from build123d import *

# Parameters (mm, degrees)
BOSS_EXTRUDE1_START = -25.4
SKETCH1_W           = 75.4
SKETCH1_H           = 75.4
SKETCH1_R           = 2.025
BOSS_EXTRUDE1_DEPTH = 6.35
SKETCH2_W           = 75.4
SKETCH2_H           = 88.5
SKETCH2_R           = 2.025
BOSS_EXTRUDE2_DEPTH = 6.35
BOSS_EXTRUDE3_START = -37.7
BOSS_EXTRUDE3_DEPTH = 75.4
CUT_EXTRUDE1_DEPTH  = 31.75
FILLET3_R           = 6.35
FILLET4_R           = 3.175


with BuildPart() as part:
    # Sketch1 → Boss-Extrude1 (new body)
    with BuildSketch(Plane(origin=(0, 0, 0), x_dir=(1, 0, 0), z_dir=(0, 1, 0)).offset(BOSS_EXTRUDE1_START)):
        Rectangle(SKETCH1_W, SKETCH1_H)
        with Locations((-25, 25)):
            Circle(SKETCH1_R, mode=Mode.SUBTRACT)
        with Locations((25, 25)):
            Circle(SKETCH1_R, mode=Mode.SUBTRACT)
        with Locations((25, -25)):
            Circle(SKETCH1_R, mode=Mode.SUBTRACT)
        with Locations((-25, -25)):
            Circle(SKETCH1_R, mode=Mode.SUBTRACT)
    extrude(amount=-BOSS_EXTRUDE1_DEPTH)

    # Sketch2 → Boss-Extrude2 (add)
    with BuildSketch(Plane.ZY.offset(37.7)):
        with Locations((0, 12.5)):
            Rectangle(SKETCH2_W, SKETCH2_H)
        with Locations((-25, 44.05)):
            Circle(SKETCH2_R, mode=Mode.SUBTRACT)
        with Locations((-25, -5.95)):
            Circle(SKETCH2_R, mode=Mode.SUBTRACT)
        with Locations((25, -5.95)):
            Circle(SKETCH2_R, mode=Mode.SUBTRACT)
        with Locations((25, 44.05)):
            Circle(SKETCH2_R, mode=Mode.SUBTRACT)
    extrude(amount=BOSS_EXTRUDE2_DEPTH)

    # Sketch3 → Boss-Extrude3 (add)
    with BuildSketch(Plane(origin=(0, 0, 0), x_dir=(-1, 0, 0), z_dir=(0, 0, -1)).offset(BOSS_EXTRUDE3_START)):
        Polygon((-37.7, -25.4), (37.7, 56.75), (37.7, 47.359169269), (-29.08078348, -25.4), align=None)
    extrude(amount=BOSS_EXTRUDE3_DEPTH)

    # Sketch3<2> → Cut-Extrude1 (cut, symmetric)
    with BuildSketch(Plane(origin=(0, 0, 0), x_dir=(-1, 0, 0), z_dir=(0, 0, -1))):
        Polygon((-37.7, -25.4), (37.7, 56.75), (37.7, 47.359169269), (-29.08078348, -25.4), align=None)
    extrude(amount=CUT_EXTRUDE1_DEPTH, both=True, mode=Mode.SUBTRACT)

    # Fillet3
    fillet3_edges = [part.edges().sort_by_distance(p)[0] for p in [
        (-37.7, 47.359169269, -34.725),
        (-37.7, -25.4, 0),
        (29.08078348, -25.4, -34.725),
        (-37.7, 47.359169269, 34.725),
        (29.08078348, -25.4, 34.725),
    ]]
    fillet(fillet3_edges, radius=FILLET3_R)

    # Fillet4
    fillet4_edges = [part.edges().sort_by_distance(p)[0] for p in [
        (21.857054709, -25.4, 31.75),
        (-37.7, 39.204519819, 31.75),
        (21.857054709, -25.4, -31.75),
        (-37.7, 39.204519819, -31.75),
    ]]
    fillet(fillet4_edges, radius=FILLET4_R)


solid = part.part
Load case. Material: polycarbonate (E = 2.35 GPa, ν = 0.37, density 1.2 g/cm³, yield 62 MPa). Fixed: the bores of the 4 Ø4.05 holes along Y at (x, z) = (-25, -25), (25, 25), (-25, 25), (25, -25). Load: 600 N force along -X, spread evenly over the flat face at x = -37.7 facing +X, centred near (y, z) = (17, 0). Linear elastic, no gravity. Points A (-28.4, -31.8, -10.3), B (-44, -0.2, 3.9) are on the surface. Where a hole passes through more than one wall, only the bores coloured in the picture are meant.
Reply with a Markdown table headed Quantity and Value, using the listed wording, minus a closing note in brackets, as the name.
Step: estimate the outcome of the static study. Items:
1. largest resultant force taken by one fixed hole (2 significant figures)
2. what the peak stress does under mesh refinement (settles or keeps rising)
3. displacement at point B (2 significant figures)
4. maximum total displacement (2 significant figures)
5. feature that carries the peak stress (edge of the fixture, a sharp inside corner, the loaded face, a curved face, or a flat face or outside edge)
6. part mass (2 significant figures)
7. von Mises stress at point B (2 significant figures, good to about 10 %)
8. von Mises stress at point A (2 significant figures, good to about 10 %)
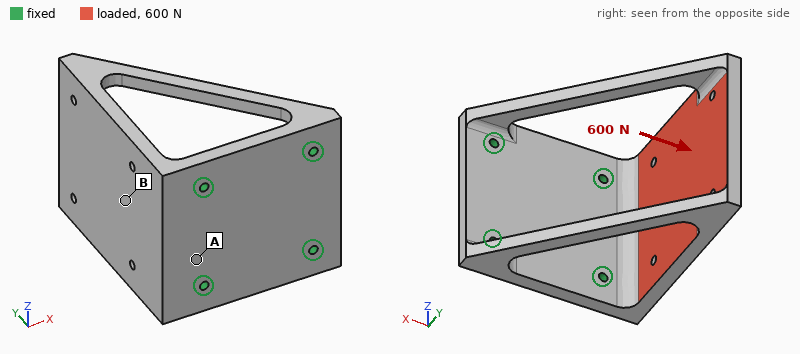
| Quantity | Value |
|---|---|
| largest resultant force taken by one fixed hole | 240 N |
| what the peak stress does under mesh refinement | keeps rising |
| displacement at point B | 0.99 mm |
| maximum total displacement | 1.5 mm |
| feature that carries the peak stress | edge of the fixture |
| part mass | 110 g |
| von Mises stress at point B | 4.3 MPa |
| von Mises stress at point A | 9.6 MPa |
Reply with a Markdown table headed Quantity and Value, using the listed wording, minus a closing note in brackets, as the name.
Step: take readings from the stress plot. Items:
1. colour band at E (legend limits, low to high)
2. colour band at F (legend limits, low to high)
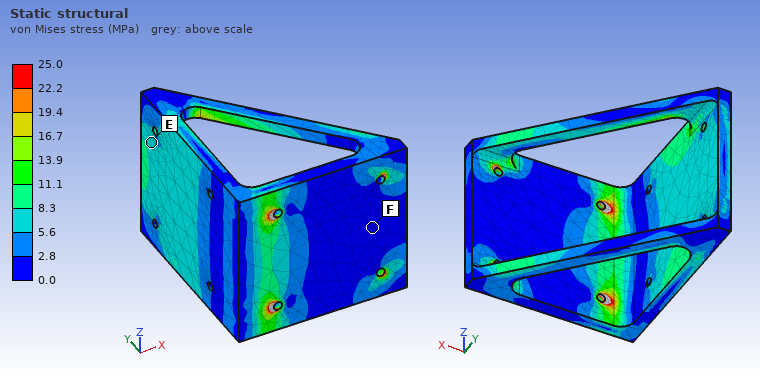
| Quantity | Value |
|---|---|
| colour band at E | 5.6 to 8.3 MPa |
| colour band at F | 0.0 to 2.8 MPa |
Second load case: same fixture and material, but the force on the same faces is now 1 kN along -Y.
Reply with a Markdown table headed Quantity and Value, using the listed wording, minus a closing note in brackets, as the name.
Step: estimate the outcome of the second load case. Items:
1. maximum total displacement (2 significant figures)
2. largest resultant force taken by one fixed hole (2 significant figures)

| Quantity | Value |
|---|---|
| maximum total displacement | 0.78 mm |
| largest resultant force taken by one fixed hole | 540 N |
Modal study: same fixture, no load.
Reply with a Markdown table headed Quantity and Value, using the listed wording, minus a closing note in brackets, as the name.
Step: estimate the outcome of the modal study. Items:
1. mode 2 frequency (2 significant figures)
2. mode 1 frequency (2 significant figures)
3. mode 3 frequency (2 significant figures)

| Quantity | Value |
|---|---|
| mode 2 frequency | 480 Hz |
| mode 1 frequency | 480 Hz |
| mode 3 frequency | 850 Hz |
